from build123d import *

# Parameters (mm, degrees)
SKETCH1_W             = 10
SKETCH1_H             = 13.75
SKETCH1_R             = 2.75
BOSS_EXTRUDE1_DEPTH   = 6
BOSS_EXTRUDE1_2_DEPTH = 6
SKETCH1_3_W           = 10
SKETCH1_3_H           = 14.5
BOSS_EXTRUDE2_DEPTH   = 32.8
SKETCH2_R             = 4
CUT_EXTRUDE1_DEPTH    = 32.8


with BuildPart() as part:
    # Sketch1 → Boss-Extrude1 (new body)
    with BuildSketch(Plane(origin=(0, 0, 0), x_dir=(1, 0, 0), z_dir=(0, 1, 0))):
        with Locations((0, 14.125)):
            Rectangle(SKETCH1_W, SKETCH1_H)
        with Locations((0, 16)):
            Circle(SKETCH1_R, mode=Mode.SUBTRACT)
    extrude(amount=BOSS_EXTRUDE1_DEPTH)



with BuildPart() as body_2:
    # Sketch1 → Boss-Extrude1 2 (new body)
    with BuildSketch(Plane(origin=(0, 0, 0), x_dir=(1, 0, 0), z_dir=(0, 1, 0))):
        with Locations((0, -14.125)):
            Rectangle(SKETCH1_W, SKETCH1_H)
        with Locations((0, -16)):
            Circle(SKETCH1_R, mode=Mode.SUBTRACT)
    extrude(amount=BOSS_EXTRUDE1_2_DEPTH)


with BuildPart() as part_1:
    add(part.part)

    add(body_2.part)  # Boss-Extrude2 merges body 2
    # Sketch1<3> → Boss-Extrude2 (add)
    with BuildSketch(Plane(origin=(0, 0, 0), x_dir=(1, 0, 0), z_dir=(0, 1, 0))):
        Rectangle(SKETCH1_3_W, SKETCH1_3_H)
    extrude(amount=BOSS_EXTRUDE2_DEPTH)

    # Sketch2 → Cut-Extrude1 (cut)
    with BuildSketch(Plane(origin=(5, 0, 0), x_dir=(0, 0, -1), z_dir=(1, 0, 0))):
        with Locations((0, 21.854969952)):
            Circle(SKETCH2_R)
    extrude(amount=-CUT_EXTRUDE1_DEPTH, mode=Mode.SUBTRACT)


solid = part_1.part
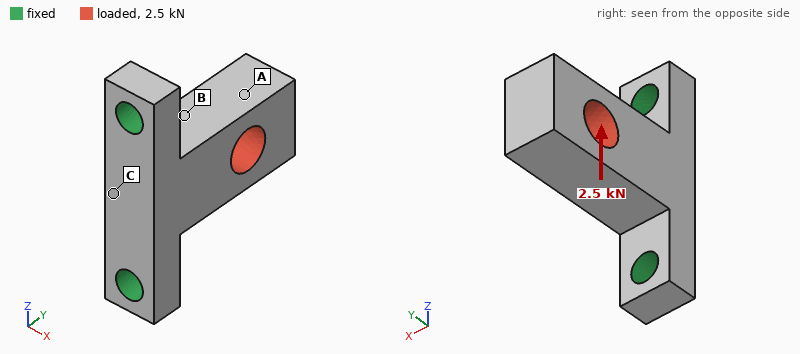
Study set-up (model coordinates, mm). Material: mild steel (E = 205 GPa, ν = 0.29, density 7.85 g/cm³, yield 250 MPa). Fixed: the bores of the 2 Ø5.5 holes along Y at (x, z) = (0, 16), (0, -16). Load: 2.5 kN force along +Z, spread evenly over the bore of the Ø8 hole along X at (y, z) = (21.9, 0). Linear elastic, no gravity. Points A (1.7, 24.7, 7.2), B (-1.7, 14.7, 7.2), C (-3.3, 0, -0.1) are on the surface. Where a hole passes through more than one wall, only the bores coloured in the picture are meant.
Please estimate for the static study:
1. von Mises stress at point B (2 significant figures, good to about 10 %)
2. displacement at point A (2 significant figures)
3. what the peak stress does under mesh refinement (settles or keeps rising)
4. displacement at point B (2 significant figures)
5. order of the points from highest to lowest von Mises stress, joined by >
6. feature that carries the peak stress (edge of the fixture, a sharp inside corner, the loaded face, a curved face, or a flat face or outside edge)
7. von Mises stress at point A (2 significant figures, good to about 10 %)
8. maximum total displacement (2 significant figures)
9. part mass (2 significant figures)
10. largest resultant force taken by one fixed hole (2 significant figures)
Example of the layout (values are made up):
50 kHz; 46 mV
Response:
70 MPa; 37 µm; keeps rising; 17 µm; B > A > C; edge of the fixture; 39 MPa; 49 µm; 44 g; 2.5 kN
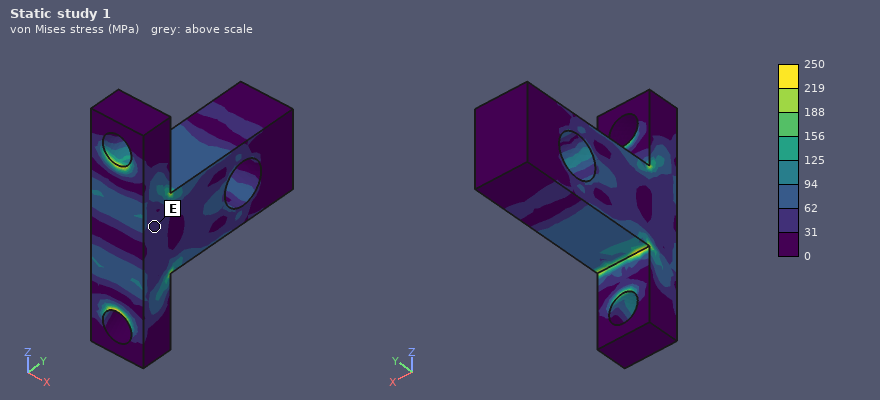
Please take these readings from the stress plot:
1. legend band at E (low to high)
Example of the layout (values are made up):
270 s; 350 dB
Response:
31 to 62 MPa
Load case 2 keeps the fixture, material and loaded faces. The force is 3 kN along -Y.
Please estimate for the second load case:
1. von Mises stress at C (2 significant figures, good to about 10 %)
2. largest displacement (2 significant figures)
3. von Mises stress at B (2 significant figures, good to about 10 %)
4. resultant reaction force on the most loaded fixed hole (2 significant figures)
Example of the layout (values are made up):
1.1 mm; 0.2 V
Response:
41 MPa; 9.0 µm; 27 MPa; 1.6 kN
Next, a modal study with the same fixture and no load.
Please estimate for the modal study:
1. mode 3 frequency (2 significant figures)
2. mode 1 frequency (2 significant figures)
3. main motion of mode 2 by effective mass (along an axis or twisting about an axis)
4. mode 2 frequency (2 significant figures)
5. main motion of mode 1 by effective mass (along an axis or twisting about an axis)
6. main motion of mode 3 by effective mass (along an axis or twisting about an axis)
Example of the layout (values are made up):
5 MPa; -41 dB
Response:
18 kHz; 4500 Hz; along Z; 9000 Hz; along X; along Y
